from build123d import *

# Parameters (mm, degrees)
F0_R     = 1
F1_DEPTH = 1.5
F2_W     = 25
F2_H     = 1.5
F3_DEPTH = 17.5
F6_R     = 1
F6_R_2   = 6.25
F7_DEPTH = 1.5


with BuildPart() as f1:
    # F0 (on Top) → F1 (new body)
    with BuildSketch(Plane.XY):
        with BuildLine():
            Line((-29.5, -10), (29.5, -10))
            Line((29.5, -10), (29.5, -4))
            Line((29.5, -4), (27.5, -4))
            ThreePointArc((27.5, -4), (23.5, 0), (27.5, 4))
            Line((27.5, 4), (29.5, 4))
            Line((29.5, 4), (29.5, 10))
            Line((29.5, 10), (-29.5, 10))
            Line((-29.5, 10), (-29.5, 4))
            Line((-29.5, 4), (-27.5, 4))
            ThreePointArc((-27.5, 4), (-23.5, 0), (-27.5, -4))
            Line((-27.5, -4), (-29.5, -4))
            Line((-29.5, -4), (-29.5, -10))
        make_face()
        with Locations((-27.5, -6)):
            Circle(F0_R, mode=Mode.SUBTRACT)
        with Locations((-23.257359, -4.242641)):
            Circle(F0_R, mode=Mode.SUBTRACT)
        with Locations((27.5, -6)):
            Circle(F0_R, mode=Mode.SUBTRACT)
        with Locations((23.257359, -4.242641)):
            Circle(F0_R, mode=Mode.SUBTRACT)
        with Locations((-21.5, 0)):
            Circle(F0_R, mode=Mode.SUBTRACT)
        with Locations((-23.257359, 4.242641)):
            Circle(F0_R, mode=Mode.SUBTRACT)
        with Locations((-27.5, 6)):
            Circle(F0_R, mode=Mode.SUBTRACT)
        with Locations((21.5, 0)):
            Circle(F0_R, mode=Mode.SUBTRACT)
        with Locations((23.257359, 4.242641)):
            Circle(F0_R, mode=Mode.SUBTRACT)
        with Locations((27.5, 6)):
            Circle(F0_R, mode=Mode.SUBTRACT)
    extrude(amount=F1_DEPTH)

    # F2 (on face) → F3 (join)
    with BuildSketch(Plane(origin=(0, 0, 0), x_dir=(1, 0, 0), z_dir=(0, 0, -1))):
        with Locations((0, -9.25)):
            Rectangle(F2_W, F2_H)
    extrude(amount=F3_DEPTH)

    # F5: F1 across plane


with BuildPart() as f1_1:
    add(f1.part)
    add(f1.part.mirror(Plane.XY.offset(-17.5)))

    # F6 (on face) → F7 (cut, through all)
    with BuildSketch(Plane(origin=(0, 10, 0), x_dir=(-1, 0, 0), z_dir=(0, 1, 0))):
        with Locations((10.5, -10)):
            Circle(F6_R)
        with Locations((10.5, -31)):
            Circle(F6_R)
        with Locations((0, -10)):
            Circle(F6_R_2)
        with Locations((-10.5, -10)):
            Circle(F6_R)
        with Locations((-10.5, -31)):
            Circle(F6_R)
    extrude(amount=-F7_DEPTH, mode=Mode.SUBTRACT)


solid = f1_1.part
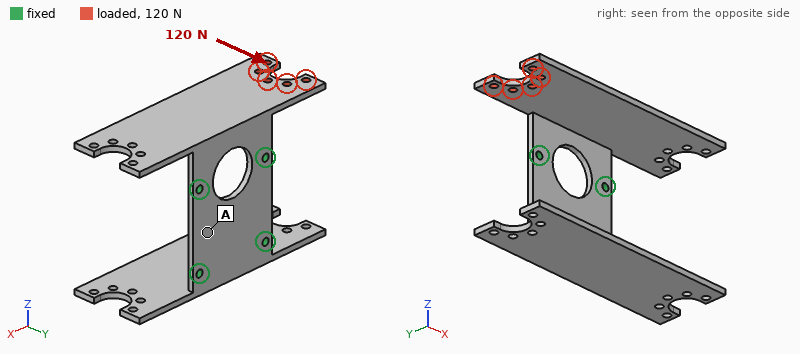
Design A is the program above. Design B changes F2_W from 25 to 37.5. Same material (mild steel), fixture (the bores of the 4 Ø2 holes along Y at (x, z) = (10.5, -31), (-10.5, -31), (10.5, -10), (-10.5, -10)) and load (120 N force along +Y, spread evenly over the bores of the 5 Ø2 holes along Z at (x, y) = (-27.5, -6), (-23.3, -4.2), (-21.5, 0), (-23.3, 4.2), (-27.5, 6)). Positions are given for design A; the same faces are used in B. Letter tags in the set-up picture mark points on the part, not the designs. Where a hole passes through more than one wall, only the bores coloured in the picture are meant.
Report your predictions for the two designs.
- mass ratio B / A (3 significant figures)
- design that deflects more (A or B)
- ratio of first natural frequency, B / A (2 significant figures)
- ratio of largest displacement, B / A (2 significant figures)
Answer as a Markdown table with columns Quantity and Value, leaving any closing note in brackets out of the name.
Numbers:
| Quantity | Value |
|---|---|
| mass ratio B / A | 1.15 |
| design that deflects more | A |
| ratio of first natural frequency, B / A | 1.3 |
| ratio of largest displacement, B / A | 0.61 |
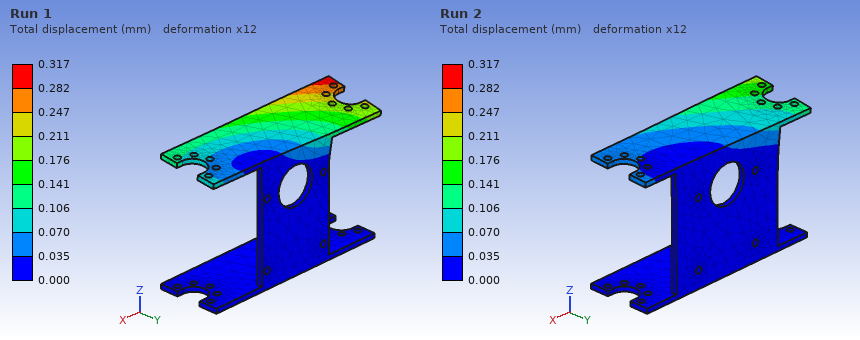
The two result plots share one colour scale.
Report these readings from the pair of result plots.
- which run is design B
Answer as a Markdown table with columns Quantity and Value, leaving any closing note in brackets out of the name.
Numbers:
| Quantity | Value |
|---|---|
| which run is design B | Run 2 |
